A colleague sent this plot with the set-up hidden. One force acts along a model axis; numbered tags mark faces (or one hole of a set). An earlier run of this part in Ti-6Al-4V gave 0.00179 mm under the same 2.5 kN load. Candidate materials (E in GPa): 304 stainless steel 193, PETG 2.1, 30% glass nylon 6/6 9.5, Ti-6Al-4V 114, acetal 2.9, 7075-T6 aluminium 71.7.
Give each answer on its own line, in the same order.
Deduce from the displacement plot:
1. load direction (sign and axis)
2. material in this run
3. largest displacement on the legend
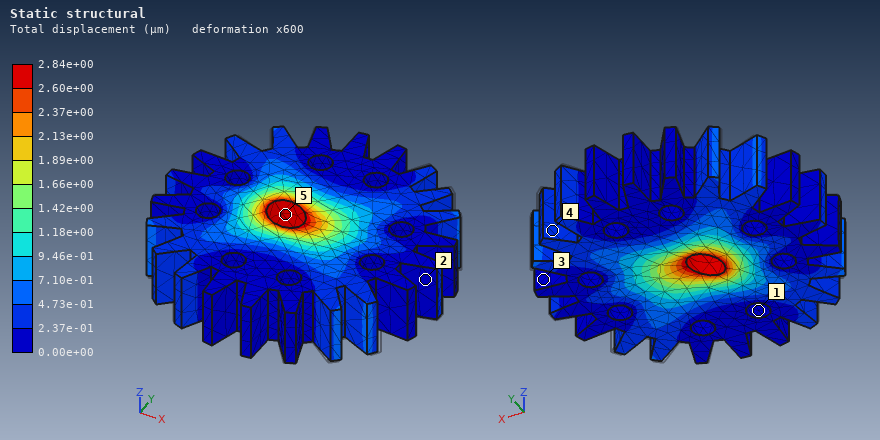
-X
7075-T6 aluminium
2.84e+00 µm
